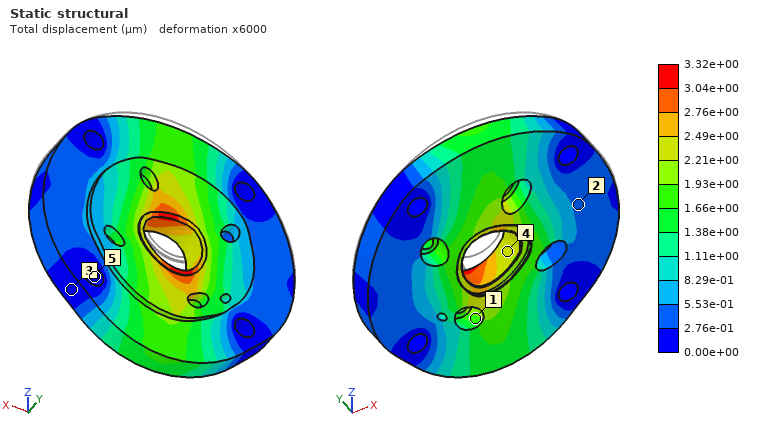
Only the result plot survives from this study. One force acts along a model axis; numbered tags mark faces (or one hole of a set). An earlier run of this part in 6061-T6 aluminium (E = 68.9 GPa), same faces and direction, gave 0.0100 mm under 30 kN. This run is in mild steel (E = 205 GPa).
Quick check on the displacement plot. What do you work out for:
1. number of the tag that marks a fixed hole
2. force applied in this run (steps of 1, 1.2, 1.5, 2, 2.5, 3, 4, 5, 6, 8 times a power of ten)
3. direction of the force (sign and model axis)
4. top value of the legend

5
30 kN
-Z
3.32e+00 µm
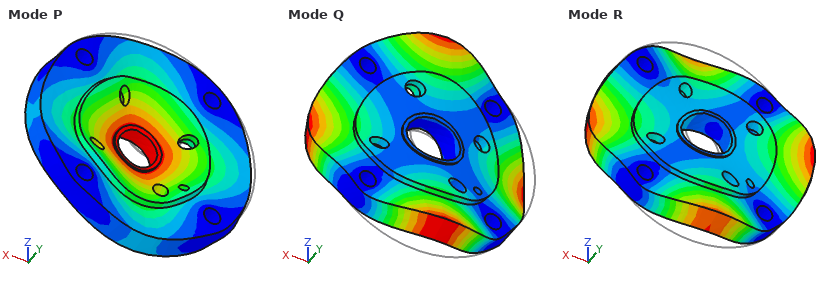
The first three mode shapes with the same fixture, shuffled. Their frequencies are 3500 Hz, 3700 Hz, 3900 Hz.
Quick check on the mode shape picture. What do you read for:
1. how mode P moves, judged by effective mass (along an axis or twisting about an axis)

along Y
